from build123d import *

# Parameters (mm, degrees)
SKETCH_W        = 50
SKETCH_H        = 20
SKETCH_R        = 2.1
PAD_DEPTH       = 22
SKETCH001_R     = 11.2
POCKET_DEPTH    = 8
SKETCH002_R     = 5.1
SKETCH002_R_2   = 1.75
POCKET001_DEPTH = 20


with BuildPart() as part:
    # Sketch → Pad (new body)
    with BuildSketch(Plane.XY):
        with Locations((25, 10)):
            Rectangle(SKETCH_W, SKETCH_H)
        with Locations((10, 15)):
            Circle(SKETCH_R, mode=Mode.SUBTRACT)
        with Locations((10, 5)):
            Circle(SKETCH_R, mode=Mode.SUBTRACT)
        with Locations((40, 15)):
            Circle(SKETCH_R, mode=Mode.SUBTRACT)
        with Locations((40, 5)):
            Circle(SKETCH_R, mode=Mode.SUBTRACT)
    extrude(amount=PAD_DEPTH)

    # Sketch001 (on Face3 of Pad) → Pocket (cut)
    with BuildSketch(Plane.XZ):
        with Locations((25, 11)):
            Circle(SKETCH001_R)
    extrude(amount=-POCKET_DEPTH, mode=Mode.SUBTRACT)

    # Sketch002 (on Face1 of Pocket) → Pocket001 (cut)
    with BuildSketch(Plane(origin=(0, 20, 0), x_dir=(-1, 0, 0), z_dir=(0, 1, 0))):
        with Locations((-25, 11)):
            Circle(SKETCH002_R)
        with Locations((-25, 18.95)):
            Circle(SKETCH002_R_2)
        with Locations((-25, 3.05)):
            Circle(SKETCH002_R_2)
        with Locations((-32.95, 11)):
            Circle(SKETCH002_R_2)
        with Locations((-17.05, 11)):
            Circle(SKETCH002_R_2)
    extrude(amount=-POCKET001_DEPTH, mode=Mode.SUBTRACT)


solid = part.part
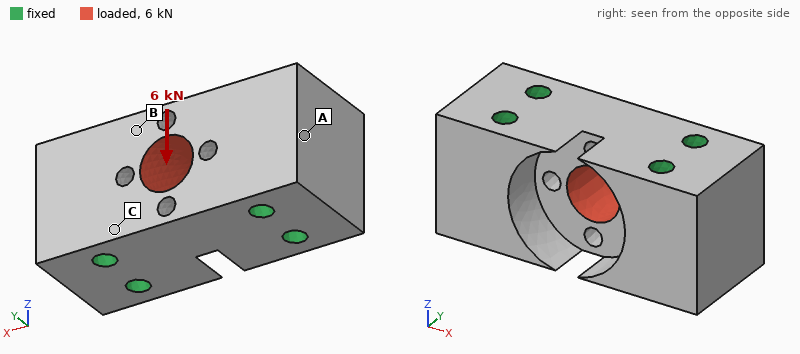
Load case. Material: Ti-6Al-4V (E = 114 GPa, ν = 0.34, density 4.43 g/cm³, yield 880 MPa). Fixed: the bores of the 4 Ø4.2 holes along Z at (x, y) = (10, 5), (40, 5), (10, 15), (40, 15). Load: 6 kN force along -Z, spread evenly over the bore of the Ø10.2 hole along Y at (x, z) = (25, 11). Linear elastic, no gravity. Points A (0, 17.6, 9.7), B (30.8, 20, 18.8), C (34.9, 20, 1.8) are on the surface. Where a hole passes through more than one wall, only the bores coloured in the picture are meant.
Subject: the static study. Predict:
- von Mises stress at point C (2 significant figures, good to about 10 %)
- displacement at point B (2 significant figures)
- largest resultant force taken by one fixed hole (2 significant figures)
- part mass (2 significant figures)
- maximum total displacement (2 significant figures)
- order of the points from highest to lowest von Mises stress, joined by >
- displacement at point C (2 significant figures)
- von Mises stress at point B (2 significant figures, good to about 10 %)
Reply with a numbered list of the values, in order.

1. 16 MPa
2. 3.5 µm
3. 2.3 kN
4. 72 g
5. 6.5 µm
6. B > C > A
7. 1.5 µm
8. 26 MPa
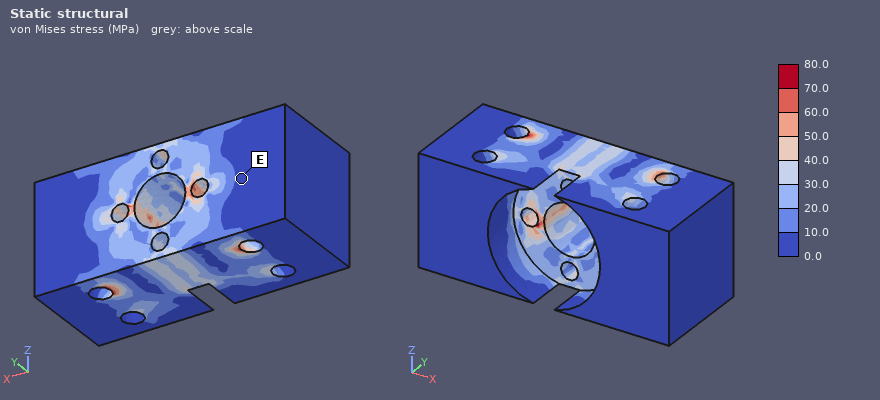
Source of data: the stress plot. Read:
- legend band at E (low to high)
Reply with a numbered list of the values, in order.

1. 0.0 to 10.0 MPa
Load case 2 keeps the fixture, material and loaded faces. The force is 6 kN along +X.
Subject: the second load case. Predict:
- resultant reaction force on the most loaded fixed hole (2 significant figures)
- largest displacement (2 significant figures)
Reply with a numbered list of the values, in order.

1. 2.4 kN
2. 2.5 µm
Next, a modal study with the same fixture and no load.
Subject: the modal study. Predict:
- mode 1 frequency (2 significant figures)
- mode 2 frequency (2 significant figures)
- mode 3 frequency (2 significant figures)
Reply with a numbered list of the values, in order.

1. 54 kHz
2. 54 kHz
3. 59 kHz
